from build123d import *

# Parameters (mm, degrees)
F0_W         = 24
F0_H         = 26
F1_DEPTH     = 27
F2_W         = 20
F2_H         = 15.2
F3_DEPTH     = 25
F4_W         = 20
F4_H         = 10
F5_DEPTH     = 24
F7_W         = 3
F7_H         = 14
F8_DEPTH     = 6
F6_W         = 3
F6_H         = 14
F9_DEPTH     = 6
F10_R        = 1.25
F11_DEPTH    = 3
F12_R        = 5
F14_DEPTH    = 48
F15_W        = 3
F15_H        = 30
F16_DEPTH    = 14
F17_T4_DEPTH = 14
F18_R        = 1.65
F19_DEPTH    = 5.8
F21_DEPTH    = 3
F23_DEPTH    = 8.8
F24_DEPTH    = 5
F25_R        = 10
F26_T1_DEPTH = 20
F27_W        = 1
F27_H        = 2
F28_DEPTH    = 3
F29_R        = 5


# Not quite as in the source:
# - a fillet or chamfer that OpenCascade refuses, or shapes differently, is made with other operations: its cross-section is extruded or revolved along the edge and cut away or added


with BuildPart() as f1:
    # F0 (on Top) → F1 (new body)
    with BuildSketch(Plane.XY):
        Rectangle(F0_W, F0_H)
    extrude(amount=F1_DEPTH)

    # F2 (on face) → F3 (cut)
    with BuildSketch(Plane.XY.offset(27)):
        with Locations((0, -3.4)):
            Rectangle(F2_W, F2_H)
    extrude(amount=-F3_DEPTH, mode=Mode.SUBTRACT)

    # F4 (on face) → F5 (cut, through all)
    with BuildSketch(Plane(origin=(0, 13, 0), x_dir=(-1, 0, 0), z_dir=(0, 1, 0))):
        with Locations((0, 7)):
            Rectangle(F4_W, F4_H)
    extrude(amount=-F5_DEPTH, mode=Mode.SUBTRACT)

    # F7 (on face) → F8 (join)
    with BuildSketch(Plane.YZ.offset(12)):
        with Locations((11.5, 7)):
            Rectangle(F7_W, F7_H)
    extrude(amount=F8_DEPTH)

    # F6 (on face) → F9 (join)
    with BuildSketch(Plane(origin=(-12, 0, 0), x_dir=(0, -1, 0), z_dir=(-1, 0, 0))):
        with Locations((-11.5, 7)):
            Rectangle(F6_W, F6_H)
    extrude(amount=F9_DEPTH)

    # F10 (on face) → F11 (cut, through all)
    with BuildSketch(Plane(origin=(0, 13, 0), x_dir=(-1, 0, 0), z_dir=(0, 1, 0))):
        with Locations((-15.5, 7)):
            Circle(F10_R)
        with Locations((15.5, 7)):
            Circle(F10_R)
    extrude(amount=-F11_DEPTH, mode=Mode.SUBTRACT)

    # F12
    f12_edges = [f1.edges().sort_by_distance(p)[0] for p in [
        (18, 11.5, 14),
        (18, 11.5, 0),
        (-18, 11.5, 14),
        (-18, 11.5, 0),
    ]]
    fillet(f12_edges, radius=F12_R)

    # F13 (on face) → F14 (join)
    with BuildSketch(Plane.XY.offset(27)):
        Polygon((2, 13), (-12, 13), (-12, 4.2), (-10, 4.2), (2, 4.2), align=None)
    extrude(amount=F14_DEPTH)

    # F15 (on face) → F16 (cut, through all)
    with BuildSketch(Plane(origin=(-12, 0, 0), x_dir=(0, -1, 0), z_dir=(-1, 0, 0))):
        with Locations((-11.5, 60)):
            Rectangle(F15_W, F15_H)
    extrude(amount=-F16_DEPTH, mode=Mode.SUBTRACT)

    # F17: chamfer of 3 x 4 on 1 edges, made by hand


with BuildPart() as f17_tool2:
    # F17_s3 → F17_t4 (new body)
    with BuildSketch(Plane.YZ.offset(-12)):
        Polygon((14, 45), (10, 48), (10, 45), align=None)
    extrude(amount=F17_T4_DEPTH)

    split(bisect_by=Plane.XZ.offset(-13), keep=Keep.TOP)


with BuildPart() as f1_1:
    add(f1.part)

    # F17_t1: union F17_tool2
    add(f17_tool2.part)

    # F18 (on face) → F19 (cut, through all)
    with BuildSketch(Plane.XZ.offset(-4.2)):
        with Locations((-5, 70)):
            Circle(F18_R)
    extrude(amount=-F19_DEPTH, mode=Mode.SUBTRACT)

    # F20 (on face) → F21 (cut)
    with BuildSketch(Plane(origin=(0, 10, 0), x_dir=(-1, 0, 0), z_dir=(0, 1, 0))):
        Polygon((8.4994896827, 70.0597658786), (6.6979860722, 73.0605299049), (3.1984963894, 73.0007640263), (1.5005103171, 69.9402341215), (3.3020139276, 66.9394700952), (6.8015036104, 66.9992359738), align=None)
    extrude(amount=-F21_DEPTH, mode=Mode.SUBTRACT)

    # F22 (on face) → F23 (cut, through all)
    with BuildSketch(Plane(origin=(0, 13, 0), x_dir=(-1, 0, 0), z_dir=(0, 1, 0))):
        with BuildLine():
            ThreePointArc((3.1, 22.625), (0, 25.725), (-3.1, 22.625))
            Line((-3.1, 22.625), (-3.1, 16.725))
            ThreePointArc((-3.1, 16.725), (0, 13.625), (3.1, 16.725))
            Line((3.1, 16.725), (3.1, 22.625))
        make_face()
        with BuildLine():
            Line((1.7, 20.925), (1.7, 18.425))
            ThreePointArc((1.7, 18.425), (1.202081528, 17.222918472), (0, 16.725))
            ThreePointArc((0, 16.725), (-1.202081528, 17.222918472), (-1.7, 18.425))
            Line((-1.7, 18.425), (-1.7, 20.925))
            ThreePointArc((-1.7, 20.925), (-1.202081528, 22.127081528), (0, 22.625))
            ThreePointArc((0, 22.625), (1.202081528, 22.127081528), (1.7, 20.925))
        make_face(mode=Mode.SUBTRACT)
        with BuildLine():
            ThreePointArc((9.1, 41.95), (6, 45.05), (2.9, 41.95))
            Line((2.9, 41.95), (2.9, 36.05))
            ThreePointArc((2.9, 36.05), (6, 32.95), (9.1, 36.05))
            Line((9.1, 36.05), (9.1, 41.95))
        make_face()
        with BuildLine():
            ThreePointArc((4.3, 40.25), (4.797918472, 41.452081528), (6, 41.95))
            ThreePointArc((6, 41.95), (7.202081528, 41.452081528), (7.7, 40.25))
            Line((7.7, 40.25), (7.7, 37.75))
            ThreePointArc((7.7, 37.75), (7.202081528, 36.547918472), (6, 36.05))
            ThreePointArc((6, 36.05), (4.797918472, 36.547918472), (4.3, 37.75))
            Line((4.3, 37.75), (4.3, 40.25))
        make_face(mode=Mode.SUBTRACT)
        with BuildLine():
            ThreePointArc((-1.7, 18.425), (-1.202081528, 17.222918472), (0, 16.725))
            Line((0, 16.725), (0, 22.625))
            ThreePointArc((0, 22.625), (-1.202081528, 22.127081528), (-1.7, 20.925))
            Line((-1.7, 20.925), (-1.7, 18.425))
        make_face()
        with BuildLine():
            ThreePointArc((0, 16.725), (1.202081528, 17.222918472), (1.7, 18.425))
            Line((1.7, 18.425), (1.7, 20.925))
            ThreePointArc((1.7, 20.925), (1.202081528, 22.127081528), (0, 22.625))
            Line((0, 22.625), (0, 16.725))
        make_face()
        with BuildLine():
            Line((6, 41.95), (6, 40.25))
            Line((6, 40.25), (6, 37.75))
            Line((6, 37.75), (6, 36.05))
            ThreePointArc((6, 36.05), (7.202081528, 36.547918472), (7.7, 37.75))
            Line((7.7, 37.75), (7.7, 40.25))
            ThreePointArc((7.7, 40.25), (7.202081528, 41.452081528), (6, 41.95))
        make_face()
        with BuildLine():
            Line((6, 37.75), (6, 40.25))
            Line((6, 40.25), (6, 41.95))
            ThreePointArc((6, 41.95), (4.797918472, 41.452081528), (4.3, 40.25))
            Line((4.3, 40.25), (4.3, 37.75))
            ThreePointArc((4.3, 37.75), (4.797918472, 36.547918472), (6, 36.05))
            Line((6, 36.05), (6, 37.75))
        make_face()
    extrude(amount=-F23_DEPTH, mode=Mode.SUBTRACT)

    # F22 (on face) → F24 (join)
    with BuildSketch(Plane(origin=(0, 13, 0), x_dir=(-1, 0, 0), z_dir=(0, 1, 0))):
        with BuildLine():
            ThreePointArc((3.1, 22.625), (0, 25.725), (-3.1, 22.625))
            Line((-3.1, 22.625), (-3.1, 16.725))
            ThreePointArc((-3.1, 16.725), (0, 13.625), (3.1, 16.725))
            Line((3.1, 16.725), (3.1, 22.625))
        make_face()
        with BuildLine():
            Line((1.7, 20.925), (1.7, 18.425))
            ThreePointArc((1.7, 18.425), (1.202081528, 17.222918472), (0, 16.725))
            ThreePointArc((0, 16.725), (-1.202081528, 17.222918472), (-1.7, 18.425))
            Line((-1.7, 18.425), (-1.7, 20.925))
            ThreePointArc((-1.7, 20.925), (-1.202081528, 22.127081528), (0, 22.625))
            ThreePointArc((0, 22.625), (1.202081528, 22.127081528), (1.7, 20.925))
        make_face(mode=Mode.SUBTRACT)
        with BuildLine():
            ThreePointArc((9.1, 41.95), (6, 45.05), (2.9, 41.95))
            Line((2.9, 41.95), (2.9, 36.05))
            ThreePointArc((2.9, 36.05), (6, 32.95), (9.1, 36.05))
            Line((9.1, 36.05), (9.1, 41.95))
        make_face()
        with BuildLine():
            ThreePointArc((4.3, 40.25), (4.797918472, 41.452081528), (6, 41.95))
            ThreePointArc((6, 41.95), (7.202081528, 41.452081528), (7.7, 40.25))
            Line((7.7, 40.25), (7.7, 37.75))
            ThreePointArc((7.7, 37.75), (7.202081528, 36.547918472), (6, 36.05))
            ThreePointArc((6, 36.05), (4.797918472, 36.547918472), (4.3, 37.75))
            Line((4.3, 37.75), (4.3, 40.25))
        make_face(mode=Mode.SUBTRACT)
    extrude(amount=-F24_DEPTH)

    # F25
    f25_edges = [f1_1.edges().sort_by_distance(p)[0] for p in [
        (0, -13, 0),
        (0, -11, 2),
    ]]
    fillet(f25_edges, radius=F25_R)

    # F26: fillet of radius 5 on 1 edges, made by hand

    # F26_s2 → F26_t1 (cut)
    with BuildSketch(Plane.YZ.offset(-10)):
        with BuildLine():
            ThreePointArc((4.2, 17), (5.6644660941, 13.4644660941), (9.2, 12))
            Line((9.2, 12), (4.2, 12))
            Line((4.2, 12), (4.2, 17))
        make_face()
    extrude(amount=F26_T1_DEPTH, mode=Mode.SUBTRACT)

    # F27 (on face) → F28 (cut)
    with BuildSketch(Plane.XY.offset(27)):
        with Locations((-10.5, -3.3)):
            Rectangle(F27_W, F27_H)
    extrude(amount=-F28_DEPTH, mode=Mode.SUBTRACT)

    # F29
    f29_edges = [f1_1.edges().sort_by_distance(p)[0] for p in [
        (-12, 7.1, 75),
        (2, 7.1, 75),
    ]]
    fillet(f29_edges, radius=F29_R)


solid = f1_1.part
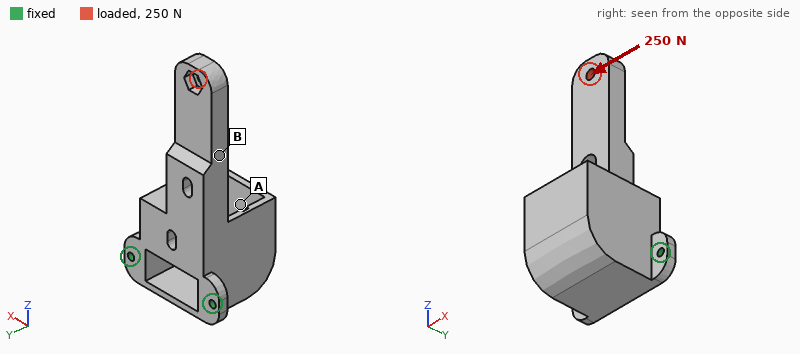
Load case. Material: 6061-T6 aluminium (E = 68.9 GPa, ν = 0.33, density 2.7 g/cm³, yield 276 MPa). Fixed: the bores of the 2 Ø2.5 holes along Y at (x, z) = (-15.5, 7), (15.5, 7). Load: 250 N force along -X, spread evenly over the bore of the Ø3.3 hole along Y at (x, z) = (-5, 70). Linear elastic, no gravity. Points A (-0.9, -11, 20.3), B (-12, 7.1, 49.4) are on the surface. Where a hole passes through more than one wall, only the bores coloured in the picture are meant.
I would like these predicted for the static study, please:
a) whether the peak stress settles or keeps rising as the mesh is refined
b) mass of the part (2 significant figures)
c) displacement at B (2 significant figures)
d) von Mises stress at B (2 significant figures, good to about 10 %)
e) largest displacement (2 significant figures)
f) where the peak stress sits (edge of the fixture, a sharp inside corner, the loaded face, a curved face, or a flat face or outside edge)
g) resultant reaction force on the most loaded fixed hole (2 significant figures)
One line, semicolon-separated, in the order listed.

keeps rising; 31 g; 0.070 mm; 27 MPa; 0.16 mm; edge of the fixture; 600 N
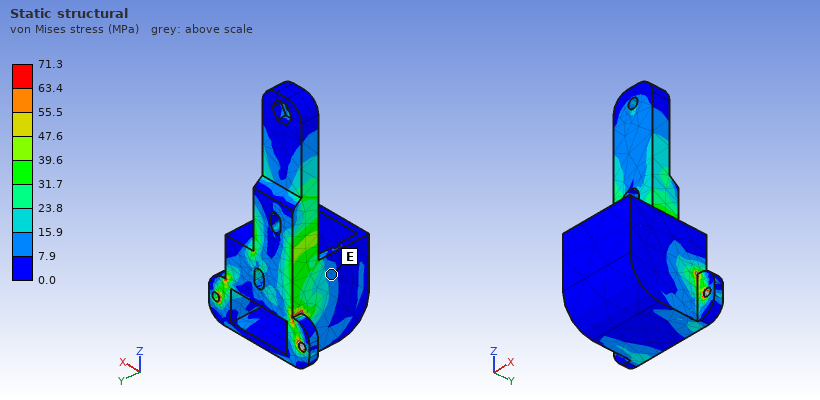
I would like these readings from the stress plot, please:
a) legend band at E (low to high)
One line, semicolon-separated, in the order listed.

7.9 to 15.9 MPa
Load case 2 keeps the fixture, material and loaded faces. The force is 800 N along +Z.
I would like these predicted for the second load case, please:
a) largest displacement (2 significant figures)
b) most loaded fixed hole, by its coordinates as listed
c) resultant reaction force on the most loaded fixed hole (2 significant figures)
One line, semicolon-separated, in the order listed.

0.38 mm; (-15.5, 7); 560 N
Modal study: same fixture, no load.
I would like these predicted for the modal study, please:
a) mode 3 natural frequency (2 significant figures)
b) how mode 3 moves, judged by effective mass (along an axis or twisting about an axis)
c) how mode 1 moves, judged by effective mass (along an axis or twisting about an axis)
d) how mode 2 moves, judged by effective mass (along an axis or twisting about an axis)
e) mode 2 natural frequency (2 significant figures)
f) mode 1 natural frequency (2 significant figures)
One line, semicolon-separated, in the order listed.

4700 Hz; along Z; along Y; along X; 3400 Hz; 980 Hz
